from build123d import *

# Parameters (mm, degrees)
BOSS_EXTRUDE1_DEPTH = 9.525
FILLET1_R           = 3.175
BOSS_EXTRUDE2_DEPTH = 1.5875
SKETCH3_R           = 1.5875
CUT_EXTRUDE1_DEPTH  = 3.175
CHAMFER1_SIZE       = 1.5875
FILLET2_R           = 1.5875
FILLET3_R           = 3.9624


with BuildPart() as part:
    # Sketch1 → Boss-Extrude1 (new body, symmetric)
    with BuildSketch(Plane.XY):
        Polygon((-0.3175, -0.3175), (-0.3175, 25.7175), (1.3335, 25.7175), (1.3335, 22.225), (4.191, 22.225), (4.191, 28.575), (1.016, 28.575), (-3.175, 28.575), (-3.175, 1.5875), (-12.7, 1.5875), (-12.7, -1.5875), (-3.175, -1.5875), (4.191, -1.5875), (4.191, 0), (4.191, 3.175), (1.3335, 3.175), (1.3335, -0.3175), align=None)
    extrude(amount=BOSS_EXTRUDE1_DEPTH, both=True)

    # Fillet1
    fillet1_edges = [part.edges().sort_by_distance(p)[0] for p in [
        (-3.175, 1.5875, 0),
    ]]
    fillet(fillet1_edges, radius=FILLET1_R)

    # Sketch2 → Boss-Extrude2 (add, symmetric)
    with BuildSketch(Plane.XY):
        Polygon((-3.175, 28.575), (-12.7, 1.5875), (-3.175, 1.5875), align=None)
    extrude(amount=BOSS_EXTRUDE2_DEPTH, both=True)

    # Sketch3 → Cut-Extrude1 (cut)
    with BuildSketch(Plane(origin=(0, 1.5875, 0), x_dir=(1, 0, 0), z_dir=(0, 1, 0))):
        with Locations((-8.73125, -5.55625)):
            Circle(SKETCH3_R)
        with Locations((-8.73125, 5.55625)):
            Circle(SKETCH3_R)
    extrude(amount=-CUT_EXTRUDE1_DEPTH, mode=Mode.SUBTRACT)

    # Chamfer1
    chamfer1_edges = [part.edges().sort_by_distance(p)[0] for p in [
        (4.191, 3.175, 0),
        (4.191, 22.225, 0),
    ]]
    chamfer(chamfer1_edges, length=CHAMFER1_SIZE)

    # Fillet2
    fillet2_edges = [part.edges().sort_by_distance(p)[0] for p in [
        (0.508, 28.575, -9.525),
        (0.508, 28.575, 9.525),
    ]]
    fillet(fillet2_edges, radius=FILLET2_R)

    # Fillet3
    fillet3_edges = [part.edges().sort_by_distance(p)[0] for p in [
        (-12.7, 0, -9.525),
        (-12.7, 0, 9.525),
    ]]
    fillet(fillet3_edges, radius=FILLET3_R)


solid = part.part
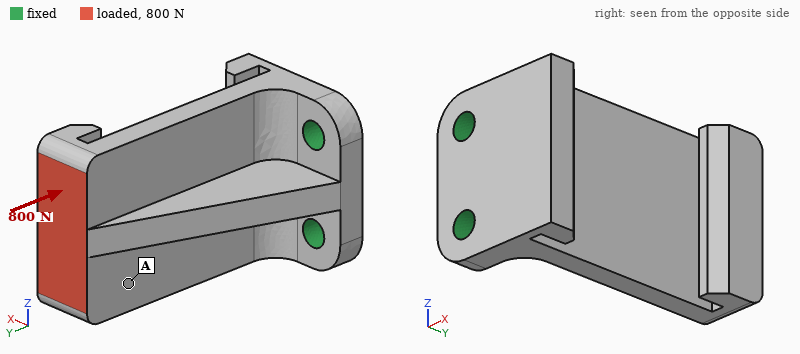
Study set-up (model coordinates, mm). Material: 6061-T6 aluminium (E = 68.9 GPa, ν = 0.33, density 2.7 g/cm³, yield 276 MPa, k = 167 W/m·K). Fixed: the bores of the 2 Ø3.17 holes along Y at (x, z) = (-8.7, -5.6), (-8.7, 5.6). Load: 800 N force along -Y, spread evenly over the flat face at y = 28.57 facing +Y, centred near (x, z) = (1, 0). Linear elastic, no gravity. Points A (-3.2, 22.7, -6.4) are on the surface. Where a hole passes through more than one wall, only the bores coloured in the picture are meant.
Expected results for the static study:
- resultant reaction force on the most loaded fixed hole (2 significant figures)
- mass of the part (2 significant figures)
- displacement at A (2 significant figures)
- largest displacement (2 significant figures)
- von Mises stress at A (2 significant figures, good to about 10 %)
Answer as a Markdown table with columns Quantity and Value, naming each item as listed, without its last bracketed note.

| Quantity | Value |
|---|---|
| resultant reaction force on the most loaded fixed hole | 400 N |
| mass of the part | 8.8 g |
| displacement at A | 0.098 mm |
| largest displacement | 0.17 mm |
| von Mises stress at A | 29 MPa |
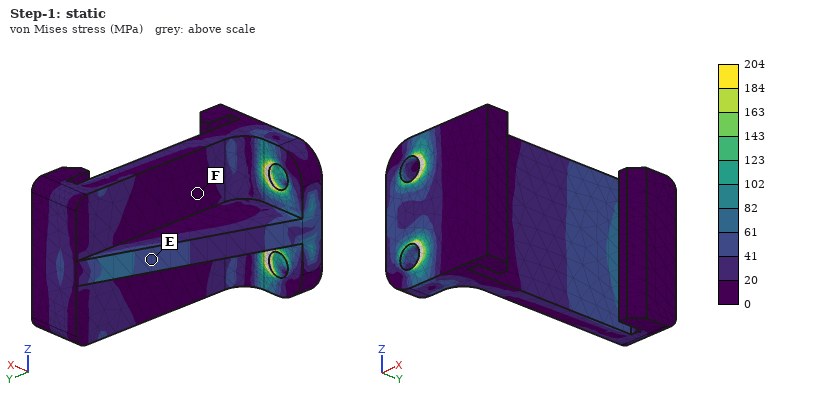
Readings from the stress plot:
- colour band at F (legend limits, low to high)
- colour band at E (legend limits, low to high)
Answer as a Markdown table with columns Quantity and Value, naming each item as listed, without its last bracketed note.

| Quantity | Value |
|---|---|
| colour band at F | 0 to 20 MPa |
| colour band at E | 41 to 61 MPa |
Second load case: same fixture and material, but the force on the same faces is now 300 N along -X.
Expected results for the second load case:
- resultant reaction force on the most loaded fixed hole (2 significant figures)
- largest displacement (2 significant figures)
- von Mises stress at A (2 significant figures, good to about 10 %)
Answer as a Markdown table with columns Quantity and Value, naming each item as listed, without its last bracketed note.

| Quantity | Value |
|---|---|
| resultant reaction force on the most loaded fixed hole | 160 N |
| largest displacement | 0.23 mm |
| von Mises stress at A | 26 MPa |
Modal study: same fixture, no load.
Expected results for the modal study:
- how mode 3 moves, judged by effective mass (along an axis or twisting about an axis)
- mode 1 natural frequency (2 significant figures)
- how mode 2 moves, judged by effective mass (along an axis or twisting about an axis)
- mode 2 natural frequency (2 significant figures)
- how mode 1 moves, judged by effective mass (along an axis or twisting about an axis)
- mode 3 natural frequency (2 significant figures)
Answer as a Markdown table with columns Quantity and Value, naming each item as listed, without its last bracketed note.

| Quantity | Value |
|---|---|
| how mode 3 moves, judged by effective mass | twisting about Y |
| mode 1 natural frequency | 3900 Hz |
| how mode 2 moves, judged by effective mass | along Z |
| mode 2 natural frequency | 6000 Hz |
| how mode 1 moves, judged by effective mass | along X |
| mode 3 natural frequency | 8200 Hz |
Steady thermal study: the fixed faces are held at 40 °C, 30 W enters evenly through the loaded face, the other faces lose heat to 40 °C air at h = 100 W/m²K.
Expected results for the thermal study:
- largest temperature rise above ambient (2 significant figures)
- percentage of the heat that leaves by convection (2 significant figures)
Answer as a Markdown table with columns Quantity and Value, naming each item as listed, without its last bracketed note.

| Quantity | Value |
|---|---|
| largest temperature rise above ambient | 72 K |
| percentage of the heat that leaves by convection | 24 % |
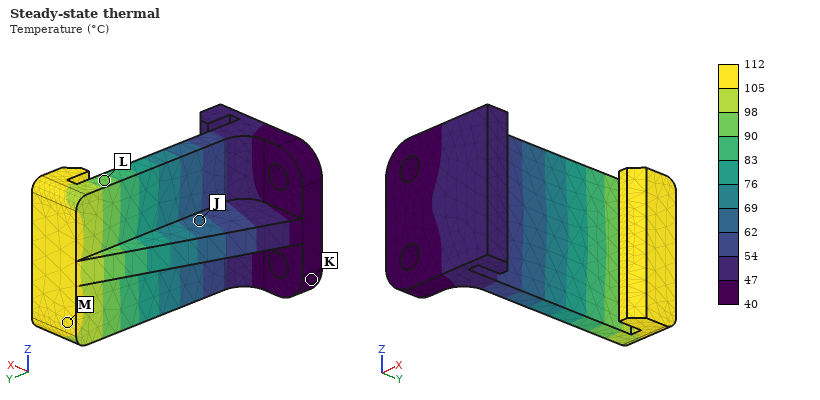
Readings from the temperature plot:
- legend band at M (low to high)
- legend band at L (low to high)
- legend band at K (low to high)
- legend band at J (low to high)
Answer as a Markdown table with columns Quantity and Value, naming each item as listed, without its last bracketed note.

| Quantity | Value |
|---|---|
| legend band at M | 105 to 112 °C |
| legend band at L | 90 to 98 °C |
| legend band at K | 40 to 47 °C |
| legend band at J | 62 to 69 °C |
